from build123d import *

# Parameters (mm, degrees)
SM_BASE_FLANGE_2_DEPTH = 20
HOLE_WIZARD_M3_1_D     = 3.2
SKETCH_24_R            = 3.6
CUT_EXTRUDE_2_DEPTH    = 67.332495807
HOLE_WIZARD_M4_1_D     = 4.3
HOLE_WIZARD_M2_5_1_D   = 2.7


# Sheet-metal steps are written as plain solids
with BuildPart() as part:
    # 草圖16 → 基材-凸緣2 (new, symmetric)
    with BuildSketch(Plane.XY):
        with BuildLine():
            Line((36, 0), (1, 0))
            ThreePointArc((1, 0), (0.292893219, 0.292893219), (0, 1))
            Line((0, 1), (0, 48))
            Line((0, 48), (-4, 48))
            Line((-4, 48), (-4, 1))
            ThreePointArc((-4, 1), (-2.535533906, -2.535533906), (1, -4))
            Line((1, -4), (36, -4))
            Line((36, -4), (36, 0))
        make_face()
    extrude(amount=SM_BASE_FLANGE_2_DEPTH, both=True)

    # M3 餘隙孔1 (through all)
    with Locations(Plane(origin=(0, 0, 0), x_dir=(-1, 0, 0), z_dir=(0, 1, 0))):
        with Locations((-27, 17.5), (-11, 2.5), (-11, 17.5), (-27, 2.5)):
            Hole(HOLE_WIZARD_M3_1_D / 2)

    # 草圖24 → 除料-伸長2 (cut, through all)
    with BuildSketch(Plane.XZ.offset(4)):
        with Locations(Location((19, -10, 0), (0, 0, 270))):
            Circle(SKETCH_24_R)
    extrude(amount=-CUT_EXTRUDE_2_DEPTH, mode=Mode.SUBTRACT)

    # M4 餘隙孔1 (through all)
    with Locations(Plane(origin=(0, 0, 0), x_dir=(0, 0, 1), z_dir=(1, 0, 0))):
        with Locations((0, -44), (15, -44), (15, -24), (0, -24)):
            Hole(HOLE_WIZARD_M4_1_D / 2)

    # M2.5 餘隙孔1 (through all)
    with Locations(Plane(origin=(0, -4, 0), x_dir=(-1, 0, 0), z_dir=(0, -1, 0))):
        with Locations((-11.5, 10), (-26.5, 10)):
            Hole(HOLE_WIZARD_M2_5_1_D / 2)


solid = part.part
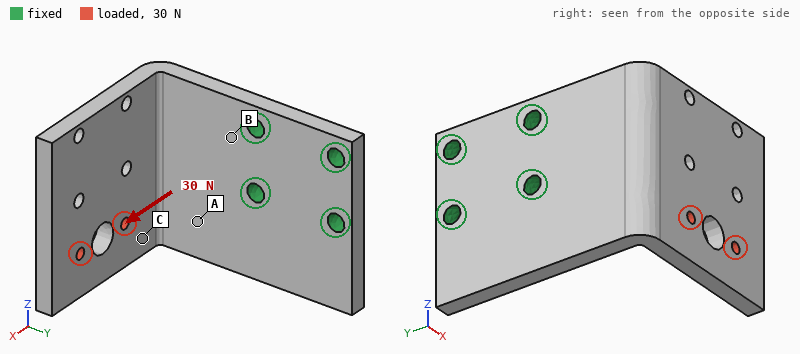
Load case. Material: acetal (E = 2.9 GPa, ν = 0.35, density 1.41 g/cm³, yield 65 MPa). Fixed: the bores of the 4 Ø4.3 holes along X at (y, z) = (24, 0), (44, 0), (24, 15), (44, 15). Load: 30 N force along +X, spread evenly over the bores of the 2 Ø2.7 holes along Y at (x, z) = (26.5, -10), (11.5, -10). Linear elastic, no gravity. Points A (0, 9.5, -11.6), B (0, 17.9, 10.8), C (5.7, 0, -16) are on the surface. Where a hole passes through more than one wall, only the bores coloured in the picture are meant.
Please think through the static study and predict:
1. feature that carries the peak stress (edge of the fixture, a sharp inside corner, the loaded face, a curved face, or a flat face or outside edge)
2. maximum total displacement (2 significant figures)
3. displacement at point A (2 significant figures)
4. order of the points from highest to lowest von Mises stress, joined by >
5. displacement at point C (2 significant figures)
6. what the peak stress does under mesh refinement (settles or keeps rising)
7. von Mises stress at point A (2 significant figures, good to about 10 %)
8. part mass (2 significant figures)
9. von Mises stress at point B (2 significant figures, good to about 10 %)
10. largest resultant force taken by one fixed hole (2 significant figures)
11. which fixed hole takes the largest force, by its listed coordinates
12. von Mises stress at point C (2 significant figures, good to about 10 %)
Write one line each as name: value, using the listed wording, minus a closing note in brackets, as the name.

feature that carries the peak stress: edge of the fixture
maximum total displacement: 0.87 mm
displacement at point A: 0.19 mm
order of the points from highest to lowest von Mises stress, joined by >: B > A > C
displacement at point C: 0.42 mm
what the peak stress does under mesh refinement: keeps rising
von Mises stress at point A: 3.0 MPa
part mass: 19 g
von Mises stress at point B: 4.7 MPa
largest resultant force taken by one fixed hole: 50 N
which fixed hole takes the largest force, by its listed coordinates: (24, 0)
von Mises stress at point C: 1.3 MPa
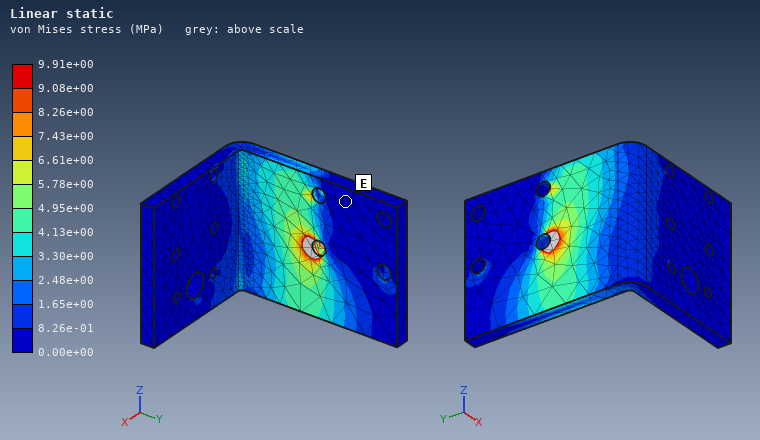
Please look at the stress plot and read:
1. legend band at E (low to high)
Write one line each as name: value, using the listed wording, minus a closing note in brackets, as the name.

legend band at E: 0.00e+00 to 8.26e-01 MPa
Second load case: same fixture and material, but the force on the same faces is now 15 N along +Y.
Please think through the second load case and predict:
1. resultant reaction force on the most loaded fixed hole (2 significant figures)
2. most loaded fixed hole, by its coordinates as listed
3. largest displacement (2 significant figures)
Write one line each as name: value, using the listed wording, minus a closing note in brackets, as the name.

resultant reaction force on the most loaded fixed hole: 15 N
most loaded fixed hole, by its coordinates as listed: (24, 0)
largest displacement: 0.73 mm
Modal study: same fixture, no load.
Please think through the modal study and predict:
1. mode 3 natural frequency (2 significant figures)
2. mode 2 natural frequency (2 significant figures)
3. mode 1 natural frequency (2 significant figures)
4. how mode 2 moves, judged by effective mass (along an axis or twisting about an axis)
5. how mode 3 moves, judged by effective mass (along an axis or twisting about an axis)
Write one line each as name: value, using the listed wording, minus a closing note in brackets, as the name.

mode 3 natural frequency: 890 Hz
mode 2 natural frequency: 500 Hz
mode 1 natural frequency: 310 Hz
how mode 2 moves, judged by effective mass: along Z
how mode 3 moves, judged by effective mass: along X
